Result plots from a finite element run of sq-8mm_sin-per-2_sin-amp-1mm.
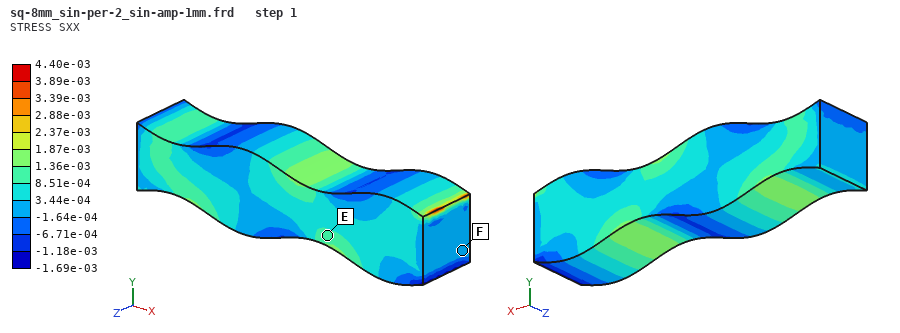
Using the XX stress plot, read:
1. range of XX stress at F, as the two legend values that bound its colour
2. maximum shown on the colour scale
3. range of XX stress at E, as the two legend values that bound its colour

-1.64e-04 to 3.44e-04
4.40e-03
8.51e-04 to 1.36e-03
